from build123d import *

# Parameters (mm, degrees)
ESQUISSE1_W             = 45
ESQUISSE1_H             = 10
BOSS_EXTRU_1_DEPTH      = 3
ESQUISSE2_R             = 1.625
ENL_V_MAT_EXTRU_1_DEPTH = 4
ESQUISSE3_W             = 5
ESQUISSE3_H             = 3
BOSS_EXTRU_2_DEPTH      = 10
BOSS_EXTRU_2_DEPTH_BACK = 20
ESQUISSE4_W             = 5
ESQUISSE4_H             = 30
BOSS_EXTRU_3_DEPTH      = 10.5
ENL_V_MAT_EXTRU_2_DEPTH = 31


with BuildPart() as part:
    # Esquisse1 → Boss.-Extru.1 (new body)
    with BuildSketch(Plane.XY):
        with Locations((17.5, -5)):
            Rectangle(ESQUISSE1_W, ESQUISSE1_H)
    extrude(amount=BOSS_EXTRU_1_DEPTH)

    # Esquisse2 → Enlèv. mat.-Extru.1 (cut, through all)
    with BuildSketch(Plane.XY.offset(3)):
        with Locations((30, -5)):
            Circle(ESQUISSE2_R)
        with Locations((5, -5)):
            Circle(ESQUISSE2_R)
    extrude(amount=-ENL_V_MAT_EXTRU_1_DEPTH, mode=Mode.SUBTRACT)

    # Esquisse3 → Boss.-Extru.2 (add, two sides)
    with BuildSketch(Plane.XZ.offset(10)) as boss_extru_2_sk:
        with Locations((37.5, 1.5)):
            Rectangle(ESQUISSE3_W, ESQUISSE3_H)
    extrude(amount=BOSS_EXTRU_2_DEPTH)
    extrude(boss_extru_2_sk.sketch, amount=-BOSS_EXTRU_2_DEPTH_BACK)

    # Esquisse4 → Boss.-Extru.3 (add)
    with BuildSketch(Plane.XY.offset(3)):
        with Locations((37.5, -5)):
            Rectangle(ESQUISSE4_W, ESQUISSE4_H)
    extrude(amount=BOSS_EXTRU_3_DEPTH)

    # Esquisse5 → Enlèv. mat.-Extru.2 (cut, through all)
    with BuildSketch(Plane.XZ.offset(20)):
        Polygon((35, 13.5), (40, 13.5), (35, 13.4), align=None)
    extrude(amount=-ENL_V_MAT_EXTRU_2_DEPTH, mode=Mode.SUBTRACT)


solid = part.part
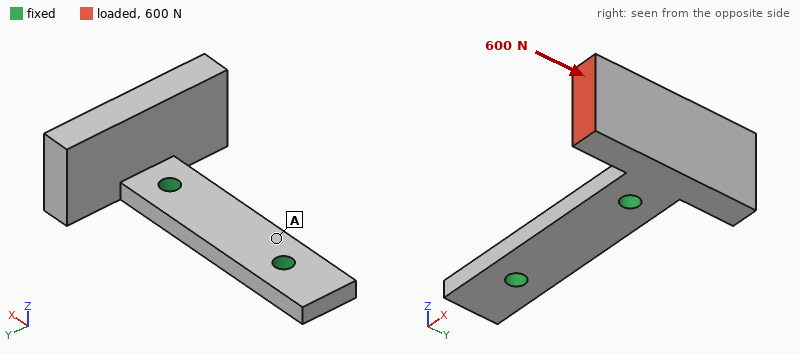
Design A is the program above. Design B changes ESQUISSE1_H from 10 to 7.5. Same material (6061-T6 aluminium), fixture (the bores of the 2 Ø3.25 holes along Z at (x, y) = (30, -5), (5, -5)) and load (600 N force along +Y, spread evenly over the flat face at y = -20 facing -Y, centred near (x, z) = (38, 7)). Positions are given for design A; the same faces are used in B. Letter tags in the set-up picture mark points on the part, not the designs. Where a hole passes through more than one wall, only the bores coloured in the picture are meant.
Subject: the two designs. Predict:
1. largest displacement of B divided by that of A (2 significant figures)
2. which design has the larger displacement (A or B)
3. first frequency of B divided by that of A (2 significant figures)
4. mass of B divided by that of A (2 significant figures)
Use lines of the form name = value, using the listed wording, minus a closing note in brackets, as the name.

largest displacement of B divided by that of A = 1.5
which design has the larger displacement = B
first frequency of B divided by that of A = 0.82
mass of B divided by that of A = 0.91
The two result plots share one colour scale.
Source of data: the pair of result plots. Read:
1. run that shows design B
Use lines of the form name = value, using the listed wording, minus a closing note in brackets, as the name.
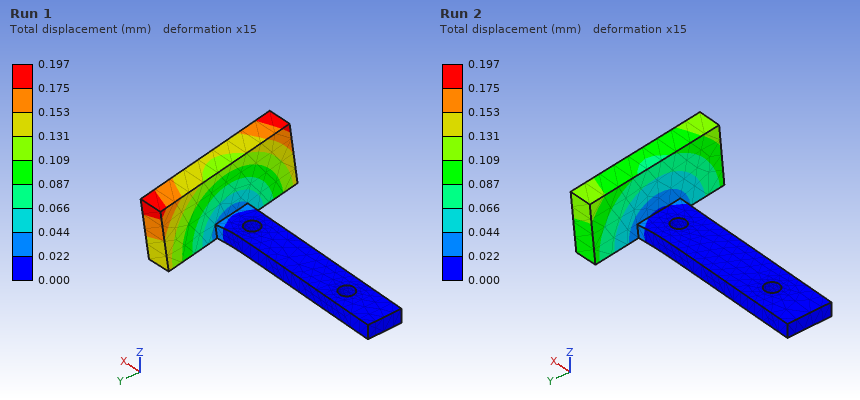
run that shows design B = Run 1
